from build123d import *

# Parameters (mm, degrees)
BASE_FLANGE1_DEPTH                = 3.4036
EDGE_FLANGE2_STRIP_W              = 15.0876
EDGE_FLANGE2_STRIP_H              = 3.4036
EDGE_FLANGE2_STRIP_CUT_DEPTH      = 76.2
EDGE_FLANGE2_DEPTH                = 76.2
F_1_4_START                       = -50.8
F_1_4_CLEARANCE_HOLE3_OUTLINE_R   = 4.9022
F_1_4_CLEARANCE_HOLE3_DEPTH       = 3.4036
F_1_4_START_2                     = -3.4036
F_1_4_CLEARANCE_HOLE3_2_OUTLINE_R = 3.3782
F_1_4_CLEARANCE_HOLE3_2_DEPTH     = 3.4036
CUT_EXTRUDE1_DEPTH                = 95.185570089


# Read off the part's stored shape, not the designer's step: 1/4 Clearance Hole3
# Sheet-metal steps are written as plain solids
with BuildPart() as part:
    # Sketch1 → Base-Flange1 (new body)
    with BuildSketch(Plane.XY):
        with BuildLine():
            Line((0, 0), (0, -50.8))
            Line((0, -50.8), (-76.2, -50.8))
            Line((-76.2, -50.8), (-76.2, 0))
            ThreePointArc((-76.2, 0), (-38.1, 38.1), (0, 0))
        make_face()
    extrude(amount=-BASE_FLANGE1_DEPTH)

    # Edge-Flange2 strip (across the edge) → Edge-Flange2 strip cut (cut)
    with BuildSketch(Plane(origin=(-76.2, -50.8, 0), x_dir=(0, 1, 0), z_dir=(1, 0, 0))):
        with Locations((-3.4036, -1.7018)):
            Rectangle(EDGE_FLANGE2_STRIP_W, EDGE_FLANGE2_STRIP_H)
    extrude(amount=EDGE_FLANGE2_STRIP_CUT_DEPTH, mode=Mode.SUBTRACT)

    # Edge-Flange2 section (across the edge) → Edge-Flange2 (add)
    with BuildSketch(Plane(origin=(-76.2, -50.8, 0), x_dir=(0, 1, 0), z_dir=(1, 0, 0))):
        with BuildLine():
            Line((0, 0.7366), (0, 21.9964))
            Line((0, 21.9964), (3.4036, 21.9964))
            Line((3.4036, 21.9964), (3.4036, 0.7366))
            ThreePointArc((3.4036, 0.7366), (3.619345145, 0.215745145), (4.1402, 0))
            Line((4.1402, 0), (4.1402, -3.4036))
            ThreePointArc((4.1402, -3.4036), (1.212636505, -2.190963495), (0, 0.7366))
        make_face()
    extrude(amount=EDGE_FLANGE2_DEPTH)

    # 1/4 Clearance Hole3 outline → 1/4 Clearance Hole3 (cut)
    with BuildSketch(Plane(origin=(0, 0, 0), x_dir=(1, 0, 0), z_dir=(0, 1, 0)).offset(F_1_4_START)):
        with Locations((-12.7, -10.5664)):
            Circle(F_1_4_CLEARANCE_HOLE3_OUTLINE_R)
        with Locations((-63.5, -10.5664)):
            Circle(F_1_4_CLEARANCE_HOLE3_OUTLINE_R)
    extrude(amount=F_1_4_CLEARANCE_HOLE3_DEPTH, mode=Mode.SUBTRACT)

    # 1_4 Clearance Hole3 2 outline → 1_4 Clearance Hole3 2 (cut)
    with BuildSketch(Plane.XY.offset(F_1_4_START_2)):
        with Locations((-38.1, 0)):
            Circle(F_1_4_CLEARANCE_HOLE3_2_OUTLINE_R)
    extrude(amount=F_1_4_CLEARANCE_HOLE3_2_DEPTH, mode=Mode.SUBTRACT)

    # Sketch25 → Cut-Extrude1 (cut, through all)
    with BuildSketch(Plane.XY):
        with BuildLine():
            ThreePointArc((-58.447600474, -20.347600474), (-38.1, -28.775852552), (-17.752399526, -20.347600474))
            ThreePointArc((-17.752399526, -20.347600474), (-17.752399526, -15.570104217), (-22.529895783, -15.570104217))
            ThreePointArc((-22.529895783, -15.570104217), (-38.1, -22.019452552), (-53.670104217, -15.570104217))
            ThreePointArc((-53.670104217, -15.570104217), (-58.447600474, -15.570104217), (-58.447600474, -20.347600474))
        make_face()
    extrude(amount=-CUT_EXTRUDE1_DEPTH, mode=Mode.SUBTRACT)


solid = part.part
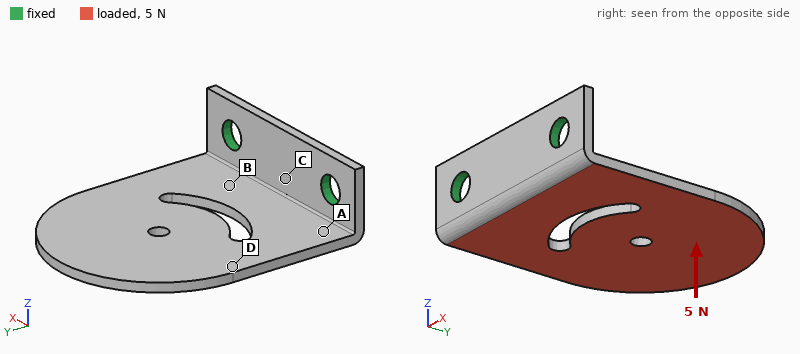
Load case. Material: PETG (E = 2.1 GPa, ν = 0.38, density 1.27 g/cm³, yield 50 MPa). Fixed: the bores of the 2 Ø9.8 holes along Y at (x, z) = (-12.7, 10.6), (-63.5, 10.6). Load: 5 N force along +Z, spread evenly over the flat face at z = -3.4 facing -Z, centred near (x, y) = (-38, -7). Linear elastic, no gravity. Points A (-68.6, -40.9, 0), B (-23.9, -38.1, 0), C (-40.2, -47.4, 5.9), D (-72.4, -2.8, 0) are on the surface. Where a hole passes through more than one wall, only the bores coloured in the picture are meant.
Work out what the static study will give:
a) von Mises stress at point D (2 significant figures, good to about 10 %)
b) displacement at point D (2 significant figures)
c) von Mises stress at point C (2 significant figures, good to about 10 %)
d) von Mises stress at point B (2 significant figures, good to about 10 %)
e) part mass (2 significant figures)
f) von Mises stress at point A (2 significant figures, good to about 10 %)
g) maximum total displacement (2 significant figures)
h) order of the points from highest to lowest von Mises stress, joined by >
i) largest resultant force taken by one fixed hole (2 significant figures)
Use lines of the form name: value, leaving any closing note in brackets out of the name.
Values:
von Mises stress at point D: 0.44 MPa
displacement at point D: 0.51 mm
von Mises stress at point C: 0.69 MPa
von Mises stress at point B: 0.97 MPa
part mass: 31 g
von Mises stress at point A: 1.2 MPa
maximum total displacement: 1.3 mm
order of the points from highest to lowest von Mises stress, joined by >: A > B > C > D
largest resultant force taken by one fixed hole: 2.5 N
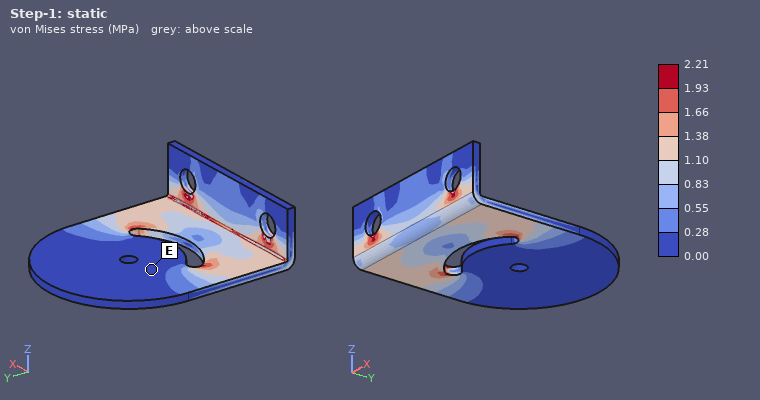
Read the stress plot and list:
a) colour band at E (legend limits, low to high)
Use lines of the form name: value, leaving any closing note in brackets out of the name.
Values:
colour band at E: 0.00 to 0.28 MPa
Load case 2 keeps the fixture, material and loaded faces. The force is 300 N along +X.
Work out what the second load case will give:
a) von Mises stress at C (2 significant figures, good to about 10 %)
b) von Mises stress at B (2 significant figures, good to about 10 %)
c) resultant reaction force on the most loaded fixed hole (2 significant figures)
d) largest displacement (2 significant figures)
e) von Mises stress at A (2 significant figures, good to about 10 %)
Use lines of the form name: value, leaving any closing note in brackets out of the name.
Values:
von Mises stress at C: 4.3 MPa
von Mises stress at B: 4.9 MPa
resultant reaction force on the most loaded fixed hole: 290 N
largest displacement: 1.1 mm
von Mises stress at A: 9.1 MPa
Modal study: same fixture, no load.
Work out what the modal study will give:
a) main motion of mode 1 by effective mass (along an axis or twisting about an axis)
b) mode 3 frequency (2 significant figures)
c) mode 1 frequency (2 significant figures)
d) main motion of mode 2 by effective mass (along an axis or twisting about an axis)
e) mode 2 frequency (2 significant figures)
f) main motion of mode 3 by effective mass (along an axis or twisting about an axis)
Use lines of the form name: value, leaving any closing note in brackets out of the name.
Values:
main motion of mode 1 by effective mass: along Z
mode 3 frequency: 480 Hz
mode 1 frequency: 84 Hz
main motion of mode 2 by effective mass: twisting about Y
mode 2 frequency: 280 Hz
main motion of mode 3 by effective mass: along Z
